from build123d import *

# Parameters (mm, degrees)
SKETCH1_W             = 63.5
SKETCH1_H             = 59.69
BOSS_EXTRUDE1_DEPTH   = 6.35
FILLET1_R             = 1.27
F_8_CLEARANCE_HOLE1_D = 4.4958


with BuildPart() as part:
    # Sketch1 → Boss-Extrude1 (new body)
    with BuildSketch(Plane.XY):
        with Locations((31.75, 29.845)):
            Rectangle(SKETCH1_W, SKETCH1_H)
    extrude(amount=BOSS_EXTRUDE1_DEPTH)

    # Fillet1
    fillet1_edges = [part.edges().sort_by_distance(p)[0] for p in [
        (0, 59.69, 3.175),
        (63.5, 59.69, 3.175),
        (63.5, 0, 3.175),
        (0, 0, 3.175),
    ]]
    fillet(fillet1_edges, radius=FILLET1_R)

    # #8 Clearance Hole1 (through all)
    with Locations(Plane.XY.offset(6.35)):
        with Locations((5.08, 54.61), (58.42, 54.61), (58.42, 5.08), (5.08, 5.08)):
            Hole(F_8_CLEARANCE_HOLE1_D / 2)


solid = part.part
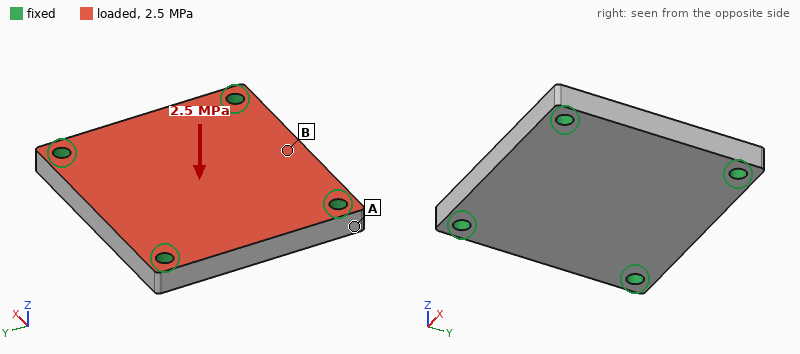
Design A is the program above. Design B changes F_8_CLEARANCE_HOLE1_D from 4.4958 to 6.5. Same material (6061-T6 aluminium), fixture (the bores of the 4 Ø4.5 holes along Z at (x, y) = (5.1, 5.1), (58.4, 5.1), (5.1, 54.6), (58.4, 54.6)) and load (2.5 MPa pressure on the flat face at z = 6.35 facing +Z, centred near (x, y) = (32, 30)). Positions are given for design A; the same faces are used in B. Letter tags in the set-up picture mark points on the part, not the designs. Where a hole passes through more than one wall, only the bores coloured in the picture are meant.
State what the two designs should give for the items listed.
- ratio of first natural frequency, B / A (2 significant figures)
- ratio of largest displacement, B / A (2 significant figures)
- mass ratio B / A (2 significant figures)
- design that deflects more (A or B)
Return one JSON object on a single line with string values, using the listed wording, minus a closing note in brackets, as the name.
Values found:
{"ratio of first natural frequency, B / A": "1.1", "ratio of largest displacement, B / A": "0.84", "mass ratio B / A": "0.98", "design that deflects more": "A"}
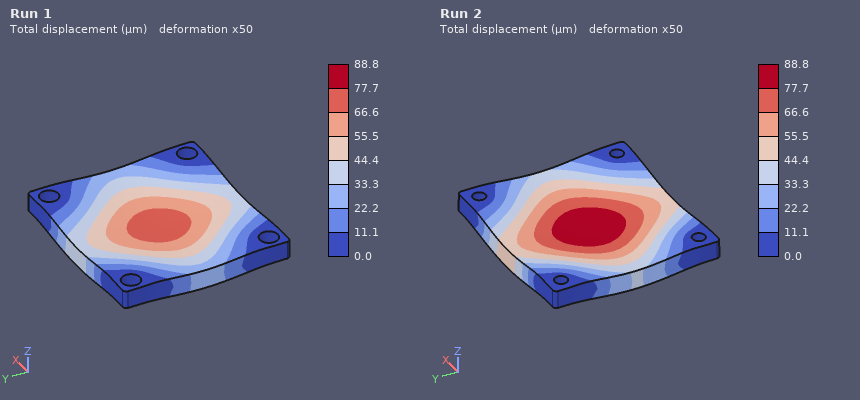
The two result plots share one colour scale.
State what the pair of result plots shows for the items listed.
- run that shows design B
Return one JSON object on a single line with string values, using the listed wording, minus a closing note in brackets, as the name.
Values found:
{"run that shows design B": "Run 1"}
